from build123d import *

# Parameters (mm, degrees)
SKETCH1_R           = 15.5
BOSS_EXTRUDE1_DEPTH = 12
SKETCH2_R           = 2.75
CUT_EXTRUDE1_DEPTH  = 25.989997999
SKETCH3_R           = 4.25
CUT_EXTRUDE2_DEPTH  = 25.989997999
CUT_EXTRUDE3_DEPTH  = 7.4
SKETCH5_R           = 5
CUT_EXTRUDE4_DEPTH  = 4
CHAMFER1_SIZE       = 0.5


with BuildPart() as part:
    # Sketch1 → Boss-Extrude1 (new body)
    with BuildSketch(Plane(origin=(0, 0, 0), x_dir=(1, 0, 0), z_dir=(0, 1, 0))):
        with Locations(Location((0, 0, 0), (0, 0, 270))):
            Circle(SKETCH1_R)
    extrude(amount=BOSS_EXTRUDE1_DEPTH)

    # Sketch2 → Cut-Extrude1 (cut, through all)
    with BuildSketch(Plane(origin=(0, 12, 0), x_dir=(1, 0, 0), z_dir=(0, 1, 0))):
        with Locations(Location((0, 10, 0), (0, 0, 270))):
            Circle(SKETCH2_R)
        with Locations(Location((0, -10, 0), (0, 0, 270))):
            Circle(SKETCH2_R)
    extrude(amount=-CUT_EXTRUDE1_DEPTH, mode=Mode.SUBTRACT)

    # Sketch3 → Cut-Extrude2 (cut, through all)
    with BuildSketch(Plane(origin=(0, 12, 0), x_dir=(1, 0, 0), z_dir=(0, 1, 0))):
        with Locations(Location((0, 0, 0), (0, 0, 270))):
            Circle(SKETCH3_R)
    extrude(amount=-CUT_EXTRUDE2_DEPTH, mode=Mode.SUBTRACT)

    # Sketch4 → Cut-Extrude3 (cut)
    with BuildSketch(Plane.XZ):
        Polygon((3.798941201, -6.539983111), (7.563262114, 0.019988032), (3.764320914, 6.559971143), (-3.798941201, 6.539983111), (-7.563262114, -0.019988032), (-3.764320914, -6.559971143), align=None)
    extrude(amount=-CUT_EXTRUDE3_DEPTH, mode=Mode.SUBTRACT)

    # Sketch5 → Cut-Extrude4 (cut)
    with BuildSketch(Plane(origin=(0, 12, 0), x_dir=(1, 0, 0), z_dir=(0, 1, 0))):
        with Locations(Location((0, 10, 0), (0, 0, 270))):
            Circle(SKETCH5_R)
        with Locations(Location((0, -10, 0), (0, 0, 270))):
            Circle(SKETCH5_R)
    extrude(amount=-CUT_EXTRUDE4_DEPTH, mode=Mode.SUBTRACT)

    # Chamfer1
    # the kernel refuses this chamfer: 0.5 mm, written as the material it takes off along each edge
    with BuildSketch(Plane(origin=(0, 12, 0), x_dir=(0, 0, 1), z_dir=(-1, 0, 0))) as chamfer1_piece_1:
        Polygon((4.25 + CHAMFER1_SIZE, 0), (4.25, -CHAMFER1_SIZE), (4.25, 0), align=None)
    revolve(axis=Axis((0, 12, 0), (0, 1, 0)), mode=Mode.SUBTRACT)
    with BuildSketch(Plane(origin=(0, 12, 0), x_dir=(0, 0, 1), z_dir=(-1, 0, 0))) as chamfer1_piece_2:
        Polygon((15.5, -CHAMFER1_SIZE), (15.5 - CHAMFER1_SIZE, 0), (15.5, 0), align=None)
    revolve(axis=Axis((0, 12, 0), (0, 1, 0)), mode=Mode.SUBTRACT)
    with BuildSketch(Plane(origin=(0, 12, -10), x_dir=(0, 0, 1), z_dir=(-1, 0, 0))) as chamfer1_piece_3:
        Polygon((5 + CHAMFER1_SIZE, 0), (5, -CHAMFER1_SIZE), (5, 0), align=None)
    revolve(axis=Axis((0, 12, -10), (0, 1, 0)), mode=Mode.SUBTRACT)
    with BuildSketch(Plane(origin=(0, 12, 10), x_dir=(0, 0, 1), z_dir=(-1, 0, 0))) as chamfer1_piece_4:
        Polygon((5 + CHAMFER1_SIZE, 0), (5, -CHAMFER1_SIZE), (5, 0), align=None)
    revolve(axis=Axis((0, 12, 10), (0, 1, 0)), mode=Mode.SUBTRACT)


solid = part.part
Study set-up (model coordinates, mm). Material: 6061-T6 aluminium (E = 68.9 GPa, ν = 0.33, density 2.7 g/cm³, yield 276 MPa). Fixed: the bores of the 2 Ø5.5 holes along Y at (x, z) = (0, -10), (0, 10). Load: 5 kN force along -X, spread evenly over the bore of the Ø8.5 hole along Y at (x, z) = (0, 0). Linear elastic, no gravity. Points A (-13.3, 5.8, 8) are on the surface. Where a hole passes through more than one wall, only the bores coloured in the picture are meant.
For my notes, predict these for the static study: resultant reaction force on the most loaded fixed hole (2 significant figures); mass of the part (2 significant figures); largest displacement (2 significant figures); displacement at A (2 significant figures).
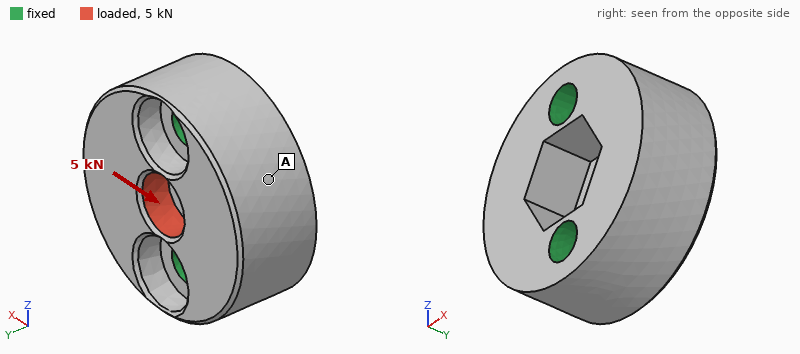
2.5 kN
18 g
21 µm
13 µm
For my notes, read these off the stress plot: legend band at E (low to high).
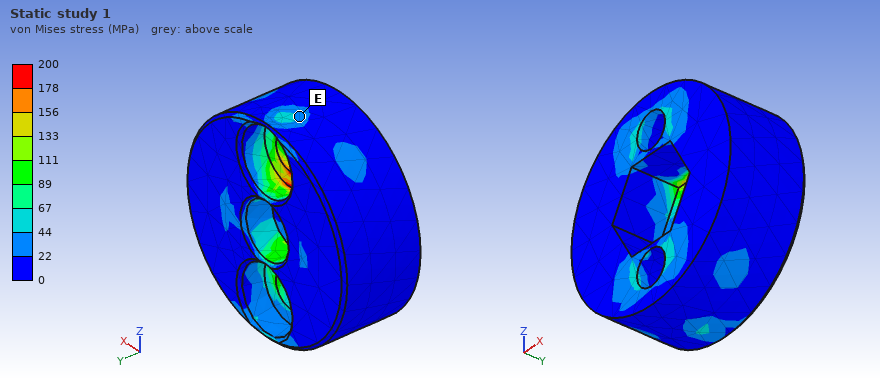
22 to 44 MPa
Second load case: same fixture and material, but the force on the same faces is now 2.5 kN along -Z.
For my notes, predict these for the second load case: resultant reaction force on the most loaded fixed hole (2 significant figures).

1.3 kN
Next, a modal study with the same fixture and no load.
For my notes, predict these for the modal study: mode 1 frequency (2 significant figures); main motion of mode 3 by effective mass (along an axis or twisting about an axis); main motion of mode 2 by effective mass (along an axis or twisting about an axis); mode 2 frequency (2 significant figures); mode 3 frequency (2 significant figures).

22 kHz
twisting about Y
along Y
26 kHz
40 kHz
